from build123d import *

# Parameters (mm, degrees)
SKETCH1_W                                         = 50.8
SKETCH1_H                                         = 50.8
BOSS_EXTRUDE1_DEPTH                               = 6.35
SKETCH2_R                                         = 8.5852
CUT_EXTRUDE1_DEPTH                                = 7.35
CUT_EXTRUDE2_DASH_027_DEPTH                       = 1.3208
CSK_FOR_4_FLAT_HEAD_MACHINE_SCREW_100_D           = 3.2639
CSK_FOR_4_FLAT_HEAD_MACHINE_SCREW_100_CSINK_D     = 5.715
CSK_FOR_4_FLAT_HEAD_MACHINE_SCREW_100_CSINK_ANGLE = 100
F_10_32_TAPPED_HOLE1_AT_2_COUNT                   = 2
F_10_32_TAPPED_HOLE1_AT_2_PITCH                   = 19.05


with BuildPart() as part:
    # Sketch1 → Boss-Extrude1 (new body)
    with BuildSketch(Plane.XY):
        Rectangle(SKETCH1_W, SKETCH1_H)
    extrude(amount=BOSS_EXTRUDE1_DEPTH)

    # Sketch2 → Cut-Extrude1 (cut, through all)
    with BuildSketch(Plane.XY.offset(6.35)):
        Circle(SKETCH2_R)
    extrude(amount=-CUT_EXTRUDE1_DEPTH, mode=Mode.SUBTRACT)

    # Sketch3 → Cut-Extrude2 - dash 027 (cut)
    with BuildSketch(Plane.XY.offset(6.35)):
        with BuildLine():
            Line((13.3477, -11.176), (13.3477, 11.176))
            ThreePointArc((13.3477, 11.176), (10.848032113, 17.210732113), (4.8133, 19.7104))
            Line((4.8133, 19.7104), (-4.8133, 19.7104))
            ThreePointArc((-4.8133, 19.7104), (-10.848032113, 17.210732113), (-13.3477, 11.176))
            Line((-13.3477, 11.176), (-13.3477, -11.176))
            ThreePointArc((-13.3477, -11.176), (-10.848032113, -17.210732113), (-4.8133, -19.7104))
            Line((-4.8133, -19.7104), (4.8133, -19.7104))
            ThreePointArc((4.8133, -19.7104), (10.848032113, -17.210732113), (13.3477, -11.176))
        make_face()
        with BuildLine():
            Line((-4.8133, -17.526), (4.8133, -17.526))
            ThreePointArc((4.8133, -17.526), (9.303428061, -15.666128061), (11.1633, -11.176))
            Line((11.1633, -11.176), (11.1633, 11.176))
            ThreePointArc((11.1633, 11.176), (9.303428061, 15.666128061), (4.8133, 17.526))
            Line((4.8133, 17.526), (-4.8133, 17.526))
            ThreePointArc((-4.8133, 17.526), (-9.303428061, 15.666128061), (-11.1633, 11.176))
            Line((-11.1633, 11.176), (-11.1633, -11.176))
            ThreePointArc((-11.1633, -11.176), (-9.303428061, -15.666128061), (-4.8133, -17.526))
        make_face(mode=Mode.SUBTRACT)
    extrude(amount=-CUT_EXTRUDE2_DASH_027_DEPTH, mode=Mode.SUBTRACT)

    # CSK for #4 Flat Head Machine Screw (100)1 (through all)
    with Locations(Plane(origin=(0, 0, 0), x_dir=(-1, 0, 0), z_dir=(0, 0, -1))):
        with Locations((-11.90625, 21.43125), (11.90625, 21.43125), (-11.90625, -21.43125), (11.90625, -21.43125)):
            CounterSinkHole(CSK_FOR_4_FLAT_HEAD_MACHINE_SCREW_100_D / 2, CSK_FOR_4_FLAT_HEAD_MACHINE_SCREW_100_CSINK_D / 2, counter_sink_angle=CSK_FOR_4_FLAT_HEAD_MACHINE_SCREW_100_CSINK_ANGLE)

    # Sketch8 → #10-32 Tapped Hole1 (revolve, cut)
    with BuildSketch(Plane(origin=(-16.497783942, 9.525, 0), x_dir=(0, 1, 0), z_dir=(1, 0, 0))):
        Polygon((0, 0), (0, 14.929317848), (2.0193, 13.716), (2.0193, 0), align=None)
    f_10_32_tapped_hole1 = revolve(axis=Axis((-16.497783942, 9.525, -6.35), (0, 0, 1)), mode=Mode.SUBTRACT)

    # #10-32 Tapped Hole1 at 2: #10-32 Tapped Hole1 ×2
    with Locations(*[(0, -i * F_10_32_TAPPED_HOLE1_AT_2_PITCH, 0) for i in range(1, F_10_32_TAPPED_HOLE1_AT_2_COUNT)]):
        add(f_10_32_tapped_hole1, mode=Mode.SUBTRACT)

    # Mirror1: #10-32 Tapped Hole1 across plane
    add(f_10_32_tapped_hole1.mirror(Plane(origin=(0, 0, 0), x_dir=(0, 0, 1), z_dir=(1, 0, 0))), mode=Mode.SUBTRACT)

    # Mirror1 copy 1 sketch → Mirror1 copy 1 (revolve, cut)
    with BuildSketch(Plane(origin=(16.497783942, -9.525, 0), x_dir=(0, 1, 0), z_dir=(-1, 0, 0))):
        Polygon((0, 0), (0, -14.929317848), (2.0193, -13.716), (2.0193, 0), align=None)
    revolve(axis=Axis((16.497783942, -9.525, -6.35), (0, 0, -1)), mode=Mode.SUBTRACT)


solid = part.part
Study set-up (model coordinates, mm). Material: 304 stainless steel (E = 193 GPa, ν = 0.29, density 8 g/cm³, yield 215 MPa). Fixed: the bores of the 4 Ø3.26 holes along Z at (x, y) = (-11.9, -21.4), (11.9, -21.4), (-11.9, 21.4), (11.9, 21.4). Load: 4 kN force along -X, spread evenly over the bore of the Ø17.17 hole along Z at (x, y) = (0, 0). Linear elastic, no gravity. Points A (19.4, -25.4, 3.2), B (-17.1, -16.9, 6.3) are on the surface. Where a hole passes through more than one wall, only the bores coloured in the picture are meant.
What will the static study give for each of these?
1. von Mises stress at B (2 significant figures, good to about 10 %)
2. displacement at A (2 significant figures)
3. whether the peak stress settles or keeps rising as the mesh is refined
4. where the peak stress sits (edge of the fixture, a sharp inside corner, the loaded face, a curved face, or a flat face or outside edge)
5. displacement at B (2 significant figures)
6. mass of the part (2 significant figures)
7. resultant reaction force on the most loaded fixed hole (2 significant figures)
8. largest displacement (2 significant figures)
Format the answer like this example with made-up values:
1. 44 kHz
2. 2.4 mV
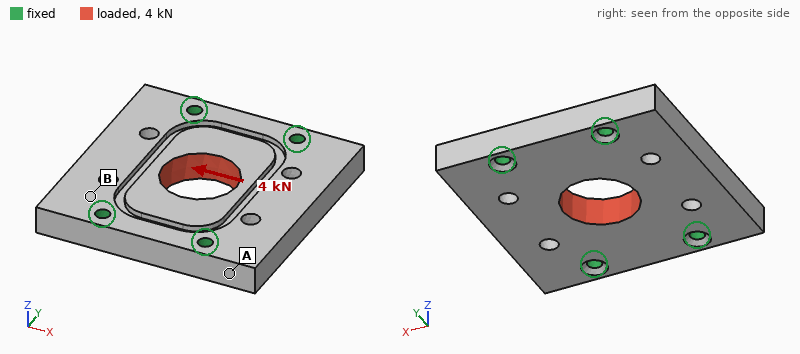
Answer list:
1. 11 MPa
2. 0.48 µm
3. keeps rising
4. edge of the fixture
5. 0.72 µm
6. 110 g
7. 1.0 kN
8. 3.0 µm
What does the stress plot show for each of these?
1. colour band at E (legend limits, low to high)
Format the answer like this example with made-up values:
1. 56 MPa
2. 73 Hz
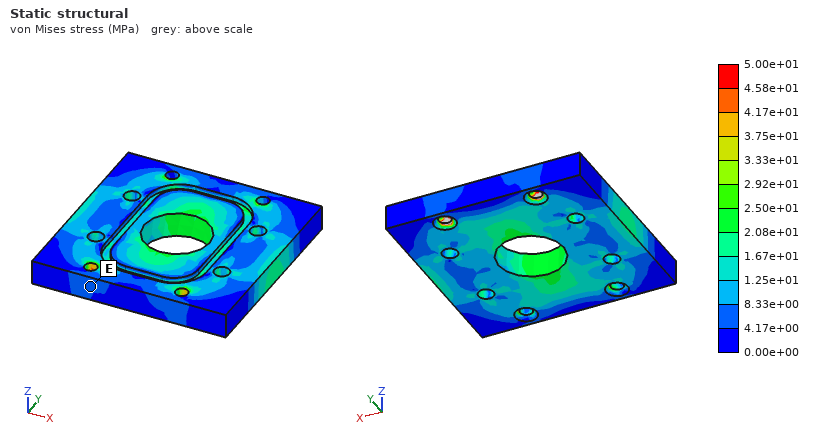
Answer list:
1. 4.17e+00 to 8.33e+00 MPa
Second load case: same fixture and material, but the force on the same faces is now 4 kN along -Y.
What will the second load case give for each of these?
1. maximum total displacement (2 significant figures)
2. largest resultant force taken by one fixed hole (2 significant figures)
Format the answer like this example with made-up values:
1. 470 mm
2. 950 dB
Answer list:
1. 1.5 µm
2. 1.0 kN
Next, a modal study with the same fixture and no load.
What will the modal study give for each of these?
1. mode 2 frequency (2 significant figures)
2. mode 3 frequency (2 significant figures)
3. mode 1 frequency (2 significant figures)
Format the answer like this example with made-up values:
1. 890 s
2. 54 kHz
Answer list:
1. 12 kHz
2. 17 kHz
3. 11 kHz
